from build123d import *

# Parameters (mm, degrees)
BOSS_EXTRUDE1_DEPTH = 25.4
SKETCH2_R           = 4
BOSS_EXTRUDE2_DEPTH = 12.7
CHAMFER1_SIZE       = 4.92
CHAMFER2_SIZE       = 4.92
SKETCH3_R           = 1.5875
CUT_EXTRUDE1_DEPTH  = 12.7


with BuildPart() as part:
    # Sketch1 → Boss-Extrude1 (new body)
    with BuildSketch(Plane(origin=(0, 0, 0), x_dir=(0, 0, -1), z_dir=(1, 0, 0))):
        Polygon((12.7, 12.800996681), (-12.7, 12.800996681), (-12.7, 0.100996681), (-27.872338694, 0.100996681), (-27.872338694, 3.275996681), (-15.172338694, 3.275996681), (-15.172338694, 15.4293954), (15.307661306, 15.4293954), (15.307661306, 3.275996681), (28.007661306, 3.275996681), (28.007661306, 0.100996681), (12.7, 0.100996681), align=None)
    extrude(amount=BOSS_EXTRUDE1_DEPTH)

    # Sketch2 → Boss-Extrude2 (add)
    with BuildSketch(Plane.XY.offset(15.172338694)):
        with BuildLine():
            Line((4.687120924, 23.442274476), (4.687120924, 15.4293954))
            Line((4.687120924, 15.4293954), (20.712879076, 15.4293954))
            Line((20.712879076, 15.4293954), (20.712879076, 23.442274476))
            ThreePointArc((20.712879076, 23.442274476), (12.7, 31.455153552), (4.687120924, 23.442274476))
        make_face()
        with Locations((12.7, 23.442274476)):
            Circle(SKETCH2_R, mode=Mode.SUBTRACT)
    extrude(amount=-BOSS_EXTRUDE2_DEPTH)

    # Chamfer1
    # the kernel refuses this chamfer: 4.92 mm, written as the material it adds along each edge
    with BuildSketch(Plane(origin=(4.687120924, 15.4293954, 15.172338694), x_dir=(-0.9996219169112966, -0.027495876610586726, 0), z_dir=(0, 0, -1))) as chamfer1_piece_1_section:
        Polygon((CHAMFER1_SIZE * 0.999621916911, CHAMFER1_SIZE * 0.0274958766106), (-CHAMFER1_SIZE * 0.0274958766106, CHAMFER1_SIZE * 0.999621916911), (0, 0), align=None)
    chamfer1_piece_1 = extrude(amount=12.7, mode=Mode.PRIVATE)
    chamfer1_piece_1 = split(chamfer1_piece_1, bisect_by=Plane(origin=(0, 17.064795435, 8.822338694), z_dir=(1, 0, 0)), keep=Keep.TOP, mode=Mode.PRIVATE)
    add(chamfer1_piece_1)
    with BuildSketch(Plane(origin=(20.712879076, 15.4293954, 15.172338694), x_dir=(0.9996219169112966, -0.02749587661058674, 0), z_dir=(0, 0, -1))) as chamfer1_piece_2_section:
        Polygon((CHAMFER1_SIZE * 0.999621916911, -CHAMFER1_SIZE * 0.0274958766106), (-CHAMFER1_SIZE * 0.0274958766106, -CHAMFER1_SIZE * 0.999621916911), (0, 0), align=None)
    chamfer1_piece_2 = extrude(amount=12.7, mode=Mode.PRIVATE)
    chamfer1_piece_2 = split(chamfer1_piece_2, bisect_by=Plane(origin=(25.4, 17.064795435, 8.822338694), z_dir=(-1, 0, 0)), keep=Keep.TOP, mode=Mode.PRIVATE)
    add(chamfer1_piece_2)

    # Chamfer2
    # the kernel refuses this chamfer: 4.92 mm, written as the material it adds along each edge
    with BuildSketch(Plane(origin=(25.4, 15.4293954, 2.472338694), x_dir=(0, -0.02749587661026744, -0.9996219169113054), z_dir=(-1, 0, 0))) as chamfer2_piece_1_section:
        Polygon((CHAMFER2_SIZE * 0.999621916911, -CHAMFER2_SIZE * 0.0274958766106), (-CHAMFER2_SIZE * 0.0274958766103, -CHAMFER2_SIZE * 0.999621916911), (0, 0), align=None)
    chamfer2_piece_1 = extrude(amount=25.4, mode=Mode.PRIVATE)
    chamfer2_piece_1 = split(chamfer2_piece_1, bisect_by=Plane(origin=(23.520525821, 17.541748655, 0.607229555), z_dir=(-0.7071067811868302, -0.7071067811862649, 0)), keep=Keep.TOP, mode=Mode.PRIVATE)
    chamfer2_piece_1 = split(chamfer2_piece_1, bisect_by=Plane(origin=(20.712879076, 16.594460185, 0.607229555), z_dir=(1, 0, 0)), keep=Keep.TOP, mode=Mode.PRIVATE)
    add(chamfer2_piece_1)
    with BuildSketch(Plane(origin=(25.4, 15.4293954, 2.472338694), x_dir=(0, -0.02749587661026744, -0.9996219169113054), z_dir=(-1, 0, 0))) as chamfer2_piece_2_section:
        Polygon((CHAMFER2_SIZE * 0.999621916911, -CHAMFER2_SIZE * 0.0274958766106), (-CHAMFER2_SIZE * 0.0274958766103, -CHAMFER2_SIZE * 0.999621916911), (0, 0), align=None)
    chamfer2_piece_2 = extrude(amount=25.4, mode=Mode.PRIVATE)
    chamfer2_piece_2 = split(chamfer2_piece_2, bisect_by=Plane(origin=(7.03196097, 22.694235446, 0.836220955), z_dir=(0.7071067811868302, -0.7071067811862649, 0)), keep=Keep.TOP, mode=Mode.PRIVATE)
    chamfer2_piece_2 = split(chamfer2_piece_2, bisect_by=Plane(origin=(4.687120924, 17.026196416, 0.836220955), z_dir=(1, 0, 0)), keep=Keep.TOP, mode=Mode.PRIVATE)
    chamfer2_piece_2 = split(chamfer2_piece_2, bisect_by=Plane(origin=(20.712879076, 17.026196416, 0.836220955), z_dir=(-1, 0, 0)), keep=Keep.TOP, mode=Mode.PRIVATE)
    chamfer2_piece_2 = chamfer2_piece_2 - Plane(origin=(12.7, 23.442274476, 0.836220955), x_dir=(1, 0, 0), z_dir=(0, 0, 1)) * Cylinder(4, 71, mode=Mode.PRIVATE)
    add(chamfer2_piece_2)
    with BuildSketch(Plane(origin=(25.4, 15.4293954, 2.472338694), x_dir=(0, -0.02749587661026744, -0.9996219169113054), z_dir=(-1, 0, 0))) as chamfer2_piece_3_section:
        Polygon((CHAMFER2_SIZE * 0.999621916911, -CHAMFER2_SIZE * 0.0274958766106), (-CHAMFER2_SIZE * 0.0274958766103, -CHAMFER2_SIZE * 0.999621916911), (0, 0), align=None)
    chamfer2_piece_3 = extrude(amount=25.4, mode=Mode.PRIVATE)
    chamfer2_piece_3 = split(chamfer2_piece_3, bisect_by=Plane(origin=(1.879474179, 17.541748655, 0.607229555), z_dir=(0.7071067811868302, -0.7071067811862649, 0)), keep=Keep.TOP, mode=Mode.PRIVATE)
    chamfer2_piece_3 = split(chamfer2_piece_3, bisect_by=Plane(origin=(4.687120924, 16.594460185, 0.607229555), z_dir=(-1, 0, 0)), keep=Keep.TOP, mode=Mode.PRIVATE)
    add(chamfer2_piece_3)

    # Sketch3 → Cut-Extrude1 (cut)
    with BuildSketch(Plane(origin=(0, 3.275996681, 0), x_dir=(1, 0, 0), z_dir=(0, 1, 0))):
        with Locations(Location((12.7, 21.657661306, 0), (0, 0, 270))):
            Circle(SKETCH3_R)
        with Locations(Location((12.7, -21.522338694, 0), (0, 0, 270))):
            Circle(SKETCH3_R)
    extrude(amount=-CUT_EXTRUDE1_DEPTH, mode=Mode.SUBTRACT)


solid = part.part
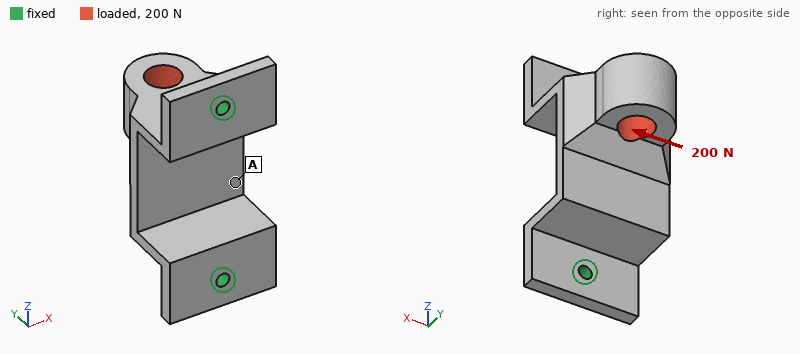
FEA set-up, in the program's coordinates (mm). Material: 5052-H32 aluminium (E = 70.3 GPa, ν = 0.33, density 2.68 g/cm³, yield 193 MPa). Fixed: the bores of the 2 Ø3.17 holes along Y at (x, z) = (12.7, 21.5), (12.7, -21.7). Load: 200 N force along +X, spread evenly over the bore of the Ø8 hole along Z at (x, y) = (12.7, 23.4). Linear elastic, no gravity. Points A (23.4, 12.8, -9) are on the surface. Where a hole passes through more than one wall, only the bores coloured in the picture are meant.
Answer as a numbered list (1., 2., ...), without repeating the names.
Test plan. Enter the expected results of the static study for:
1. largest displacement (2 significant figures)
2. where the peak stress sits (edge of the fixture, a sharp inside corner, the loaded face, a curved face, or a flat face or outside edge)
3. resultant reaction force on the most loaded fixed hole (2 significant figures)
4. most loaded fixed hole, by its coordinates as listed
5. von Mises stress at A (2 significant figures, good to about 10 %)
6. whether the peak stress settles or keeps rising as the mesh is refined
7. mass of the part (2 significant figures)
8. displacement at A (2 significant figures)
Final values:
1. 100 µm
2. edge of the fixture
3. 130 N
4. (12.7, 21.5)
5. 14 MPa
6. keeps rising
7. 23 g
8. 38 µm
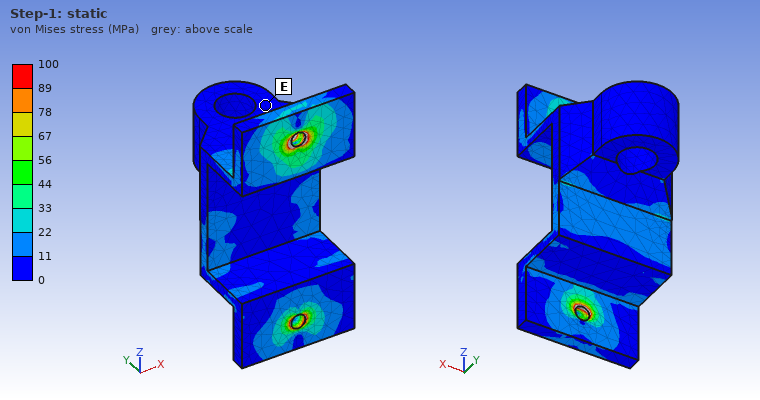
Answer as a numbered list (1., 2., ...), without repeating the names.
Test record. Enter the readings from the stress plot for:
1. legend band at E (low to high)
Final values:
1. 0 to 11 MPa
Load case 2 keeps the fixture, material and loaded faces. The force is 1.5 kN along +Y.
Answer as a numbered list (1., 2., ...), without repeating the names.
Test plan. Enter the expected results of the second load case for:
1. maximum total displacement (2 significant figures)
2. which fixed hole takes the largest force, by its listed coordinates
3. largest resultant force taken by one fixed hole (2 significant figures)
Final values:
1. 46 µm
2. (12.7, 21.5)
3. 1.2 kN
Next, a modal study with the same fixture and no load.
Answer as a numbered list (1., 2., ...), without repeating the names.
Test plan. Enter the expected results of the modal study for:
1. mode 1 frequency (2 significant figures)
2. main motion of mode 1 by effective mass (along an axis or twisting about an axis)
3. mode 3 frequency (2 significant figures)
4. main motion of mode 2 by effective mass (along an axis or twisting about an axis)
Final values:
1. 2700 Hz
2. along X
3. 8300 Hz
4. along Z
